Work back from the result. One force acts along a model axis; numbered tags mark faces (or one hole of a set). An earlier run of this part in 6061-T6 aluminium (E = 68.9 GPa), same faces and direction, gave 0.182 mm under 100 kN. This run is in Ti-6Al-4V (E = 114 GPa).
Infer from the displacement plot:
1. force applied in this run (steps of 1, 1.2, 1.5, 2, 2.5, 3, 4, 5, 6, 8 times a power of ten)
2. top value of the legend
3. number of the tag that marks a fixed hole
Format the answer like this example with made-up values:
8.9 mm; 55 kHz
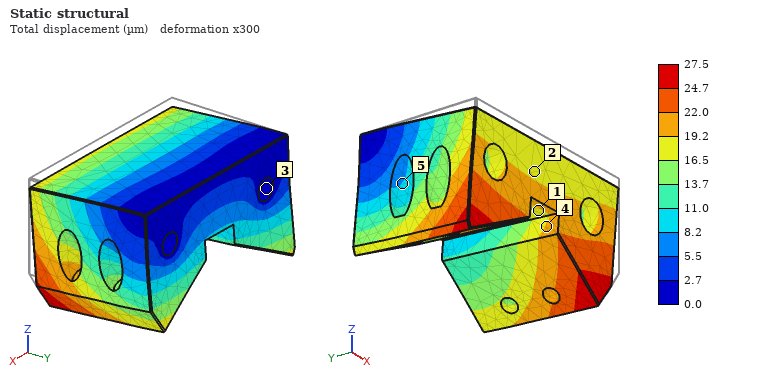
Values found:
25 kN; 27.5 µm; 3
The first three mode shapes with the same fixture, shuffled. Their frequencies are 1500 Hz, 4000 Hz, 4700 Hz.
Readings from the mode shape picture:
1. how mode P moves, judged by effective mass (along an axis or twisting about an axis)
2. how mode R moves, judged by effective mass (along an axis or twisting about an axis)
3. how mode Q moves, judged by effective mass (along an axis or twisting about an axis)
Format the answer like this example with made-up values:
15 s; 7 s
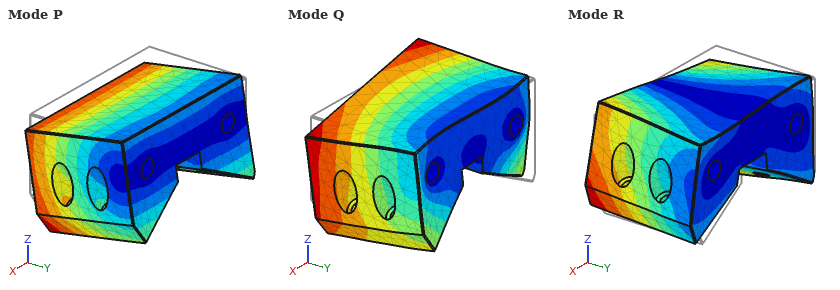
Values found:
along Z; along X; along X
